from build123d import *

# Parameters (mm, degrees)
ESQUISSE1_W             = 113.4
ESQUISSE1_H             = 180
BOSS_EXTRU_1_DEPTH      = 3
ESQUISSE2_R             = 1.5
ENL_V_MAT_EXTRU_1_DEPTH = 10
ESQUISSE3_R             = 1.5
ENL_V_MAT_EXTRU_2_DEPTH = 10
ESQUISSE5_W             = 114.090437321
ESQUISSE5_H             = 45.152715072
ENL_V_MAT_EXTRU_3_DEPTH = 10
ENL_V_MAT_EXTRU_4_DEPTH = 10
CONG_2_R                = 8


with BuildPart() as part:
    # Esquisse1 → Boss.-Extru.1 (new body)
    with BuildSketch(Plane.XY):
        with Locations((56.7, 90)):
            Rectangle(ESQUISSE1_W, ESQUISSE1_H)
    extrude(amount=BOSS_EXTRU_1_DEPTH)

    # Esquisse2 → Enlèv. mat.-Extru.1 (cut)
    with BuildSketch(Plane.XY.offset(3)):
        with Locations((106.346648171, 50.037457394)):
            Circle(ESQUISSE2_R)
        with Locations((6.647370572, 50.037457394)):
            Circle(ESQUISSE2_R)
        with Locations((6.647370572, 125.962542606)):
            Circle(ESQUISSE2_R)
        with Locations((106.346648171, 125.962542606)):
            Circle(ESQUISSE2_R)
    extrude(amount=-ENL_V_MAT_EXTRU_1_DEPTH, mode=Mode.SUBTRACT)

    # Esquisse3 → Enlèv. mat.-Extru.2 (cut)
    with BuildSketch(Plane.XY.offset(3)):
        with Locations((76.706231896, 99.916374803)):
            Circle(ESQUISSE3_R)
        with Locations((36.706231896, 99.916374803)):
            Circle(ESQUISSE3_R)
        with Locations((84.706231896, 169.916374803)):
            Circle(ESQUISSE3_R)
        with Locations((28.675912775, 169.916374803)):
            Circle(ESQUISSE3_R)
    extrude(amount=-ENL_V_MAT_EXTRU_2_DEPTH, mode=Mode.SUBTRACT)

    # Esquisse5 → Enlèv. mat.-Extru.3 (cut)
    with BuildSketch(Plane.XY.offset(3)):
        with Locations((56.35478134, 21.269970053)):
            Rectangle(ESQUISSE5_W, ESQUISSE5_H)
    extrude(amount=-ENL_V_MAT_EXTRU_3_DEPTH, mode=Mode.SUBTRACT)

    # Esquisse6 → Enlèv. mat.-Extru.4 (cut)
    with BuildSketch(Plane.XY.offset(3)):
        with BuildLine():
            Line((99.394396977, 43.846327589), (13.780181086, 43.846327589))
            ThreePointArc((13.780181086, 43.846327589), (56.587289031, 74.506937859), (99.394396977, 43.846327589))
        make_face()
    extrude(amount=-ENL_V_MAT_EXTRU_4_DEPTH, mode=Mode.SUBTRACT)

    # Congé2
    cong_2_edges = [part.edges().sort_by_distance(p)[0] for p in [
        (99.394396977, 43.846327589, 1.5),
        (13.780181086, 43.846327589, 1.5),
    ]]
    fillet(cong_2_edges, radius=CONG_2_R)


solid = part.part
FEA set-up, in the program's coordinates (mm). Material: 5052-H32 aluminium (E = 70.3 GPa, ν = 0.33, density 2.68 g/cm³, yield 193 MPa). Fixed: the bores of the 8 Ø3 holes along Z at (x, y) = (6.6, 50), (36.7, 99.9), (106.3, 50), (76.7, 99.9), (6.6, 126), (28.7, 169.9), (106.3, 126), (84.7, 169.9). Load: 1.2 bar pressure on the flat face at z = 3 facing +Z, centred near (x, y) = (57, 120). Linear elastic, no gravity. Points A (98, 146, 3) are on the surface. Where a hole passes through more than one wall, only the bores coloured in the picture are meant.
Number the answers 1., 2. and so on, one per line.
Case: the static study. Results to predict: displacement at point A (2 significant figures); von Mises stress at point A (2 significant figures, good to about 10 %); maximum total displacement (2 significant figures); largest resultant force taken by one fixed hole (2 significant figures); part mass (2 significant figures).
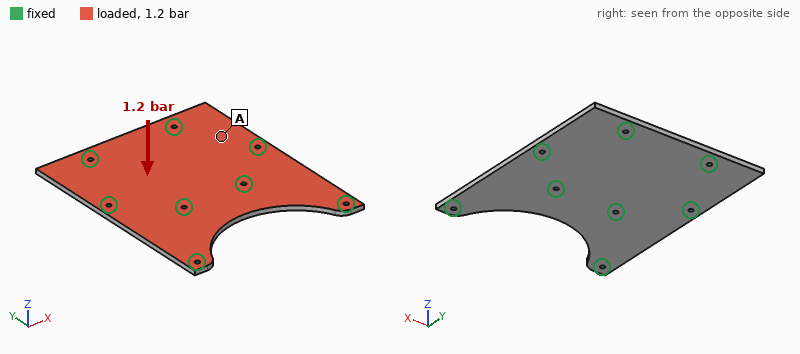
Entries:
1. 20 µm
2. 13 MPa
3. 52 µm
4. 290 N
5. 110 g
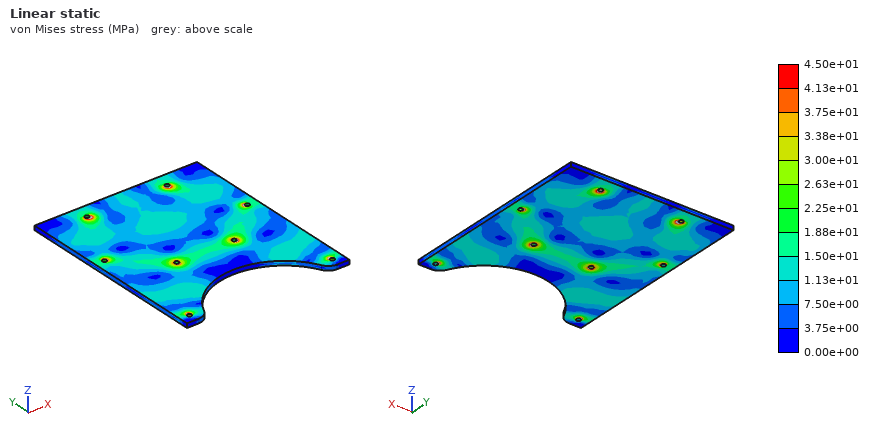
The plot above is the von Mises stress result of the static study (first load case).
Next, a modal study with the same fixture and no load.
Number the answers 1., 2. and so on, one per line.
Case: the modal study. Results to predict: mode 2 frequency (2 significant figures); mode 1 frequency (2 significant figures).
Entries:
1. 3400 Hz
2. 2900 Hz
